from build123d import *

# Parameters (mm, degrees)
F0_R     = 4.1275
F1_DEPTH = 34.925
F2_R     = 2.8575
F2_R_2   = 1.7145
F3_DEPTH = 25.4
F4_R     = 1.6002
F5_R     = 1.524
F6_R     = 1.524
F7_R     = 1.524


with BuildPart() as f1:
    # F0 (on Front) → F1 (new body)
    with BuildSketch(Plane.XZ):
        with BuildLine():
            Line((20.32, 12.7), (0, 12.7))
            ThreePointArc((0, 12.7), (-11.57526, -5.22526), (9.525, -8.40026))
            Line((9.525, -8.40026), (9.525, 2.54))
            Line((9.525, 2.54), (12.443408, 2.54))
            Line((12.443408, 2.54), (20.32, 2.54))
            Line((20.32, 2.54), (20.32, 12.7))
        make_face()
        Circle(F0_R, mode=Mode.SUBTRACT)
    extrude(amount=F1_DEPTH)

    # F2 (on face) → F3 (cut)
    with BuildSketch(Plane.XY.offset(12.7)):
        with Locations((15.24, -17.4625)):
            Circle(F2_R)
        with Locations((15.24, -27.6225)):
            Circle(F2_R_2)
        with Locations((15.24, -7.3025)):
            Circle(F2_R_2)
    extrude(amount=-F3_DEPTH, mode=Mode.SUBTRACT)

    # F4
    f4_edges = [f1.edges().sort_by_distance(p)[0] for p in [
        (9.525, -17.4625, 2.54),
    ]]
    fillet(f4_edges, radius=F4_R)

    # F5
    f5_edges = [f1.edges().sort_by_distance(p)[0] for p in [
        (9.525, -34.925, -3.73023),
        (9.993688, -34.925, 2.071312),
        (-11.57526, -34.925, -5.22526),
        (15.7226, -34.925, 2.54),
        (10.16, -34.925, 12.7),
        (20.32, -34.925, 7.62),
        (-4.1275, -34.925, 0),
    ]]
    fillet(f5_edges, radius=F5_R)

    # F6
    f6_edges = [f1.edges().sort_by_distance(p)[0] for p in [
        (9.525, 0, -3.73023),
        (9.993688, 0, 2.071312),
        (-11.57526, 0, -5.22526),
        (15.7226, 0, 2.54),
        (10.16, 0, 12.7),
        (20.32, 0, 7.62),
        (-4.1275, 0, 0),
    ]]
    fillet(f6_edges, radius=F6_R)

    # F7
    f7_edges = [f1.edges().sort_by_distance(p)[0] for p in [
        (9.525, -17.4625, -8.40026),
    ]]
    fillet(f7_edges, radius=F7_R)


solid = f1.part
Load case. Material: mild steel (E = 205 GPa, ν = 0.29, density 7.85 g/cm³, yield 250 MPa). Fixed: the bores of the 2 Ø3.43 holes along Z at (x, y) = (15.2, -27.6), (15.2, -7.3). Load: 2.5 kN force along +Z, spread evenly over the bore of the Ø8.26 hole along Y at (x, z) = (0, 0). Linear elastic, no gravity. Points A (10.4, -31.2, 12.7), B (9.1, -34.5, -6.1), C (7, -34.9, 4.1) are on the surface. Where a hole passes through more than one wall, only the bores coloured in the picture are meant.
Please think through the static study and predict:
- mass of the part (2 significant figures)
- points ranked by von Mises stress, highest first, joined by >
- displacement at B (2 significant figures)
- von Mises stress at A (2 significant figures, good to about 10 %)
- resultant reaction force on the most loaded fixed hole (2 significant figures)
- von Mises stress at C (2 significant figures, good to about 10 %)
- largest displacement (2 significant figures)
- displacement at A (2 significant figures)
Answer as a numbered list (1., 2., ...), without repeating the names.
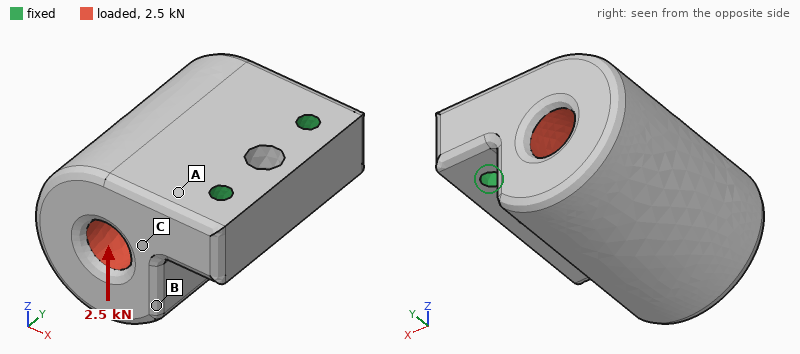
1. 140 g
2. A > C > B
3. 8.3 µm
4. 42 MPa
5. 1.3 kN
6. 26 MPa
7. 17 µm
8. 2.6 µm
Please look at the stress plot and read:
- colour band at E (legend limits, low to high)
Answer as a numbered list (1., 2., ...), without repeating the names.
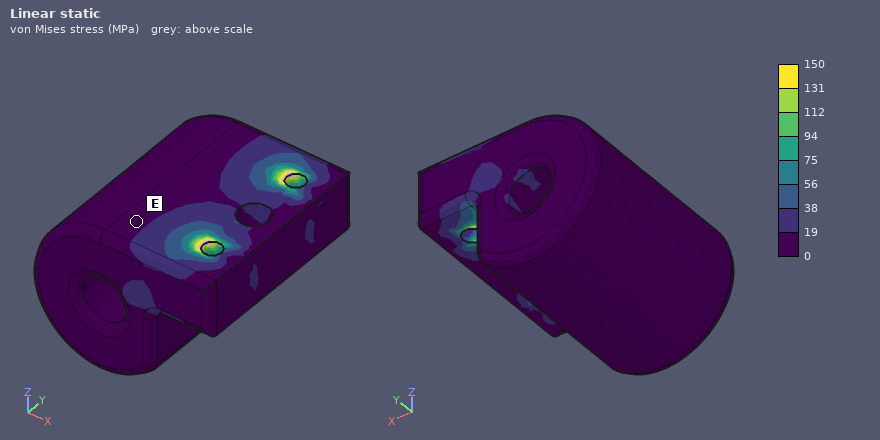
1. 0 to 19 MPa
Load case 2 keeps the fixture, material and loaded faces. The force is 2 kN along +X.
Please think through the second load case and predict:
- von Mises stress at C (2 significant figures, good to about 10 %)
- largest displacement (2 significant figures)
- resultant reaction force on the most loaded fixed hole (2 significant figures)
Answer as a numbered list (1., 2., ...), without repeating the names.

1. 15 MPa
2. 8.6 µm
3. 1.0 kN
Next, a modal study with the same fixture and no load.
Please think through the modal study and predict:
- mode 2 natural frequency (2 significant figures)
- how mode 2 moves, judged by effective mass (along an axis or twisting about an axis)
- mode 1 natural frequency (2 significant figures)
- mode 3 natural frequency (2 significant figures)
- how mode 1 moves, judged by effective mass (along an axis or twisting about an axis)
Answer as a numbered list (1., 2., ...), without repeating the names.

1. 12 kHz
2. along Y
3. 5800 Hz
4. 16 kHz
5. along Z
